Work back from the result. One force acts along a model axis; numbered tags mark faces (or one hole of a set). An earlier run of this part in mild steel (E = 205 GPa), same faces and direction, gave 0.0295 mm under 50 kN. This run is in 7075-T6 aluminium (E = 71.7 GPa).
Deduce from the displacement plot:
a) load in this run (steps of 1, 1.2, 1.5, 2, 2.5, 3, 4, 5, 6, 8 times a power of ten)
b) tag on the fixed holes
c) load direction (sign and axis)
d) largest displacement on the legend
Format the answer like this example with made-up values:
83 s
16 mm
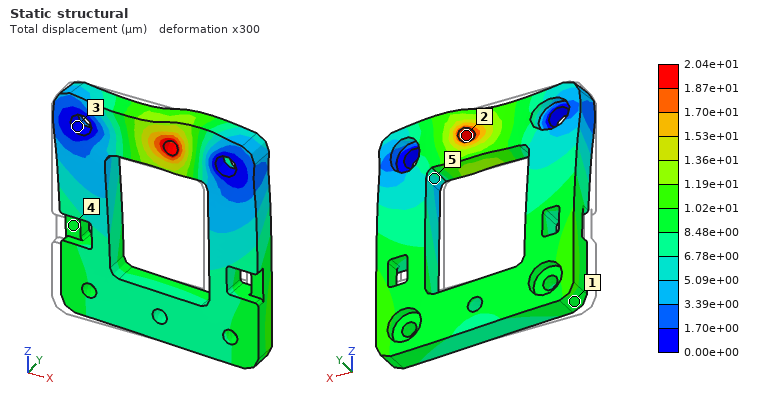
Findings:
12 kN
3
+X
2.04e+01 µm
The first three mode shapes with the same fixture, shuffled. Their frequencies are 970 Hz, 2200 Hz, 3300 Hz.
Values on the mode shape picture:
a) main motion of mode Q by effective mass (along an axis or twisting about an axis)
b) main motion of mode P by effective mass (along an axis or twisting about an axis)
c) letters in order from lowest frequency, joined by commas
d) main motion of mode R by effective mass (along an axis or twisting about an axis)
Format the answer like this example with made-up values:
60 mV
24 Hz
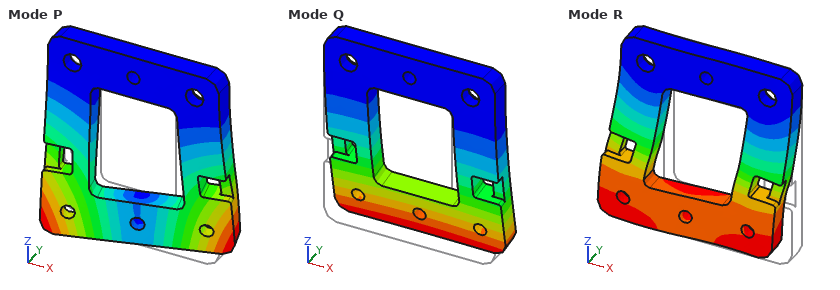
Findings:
along Y
twisting about Z
Q, P, R
along X
